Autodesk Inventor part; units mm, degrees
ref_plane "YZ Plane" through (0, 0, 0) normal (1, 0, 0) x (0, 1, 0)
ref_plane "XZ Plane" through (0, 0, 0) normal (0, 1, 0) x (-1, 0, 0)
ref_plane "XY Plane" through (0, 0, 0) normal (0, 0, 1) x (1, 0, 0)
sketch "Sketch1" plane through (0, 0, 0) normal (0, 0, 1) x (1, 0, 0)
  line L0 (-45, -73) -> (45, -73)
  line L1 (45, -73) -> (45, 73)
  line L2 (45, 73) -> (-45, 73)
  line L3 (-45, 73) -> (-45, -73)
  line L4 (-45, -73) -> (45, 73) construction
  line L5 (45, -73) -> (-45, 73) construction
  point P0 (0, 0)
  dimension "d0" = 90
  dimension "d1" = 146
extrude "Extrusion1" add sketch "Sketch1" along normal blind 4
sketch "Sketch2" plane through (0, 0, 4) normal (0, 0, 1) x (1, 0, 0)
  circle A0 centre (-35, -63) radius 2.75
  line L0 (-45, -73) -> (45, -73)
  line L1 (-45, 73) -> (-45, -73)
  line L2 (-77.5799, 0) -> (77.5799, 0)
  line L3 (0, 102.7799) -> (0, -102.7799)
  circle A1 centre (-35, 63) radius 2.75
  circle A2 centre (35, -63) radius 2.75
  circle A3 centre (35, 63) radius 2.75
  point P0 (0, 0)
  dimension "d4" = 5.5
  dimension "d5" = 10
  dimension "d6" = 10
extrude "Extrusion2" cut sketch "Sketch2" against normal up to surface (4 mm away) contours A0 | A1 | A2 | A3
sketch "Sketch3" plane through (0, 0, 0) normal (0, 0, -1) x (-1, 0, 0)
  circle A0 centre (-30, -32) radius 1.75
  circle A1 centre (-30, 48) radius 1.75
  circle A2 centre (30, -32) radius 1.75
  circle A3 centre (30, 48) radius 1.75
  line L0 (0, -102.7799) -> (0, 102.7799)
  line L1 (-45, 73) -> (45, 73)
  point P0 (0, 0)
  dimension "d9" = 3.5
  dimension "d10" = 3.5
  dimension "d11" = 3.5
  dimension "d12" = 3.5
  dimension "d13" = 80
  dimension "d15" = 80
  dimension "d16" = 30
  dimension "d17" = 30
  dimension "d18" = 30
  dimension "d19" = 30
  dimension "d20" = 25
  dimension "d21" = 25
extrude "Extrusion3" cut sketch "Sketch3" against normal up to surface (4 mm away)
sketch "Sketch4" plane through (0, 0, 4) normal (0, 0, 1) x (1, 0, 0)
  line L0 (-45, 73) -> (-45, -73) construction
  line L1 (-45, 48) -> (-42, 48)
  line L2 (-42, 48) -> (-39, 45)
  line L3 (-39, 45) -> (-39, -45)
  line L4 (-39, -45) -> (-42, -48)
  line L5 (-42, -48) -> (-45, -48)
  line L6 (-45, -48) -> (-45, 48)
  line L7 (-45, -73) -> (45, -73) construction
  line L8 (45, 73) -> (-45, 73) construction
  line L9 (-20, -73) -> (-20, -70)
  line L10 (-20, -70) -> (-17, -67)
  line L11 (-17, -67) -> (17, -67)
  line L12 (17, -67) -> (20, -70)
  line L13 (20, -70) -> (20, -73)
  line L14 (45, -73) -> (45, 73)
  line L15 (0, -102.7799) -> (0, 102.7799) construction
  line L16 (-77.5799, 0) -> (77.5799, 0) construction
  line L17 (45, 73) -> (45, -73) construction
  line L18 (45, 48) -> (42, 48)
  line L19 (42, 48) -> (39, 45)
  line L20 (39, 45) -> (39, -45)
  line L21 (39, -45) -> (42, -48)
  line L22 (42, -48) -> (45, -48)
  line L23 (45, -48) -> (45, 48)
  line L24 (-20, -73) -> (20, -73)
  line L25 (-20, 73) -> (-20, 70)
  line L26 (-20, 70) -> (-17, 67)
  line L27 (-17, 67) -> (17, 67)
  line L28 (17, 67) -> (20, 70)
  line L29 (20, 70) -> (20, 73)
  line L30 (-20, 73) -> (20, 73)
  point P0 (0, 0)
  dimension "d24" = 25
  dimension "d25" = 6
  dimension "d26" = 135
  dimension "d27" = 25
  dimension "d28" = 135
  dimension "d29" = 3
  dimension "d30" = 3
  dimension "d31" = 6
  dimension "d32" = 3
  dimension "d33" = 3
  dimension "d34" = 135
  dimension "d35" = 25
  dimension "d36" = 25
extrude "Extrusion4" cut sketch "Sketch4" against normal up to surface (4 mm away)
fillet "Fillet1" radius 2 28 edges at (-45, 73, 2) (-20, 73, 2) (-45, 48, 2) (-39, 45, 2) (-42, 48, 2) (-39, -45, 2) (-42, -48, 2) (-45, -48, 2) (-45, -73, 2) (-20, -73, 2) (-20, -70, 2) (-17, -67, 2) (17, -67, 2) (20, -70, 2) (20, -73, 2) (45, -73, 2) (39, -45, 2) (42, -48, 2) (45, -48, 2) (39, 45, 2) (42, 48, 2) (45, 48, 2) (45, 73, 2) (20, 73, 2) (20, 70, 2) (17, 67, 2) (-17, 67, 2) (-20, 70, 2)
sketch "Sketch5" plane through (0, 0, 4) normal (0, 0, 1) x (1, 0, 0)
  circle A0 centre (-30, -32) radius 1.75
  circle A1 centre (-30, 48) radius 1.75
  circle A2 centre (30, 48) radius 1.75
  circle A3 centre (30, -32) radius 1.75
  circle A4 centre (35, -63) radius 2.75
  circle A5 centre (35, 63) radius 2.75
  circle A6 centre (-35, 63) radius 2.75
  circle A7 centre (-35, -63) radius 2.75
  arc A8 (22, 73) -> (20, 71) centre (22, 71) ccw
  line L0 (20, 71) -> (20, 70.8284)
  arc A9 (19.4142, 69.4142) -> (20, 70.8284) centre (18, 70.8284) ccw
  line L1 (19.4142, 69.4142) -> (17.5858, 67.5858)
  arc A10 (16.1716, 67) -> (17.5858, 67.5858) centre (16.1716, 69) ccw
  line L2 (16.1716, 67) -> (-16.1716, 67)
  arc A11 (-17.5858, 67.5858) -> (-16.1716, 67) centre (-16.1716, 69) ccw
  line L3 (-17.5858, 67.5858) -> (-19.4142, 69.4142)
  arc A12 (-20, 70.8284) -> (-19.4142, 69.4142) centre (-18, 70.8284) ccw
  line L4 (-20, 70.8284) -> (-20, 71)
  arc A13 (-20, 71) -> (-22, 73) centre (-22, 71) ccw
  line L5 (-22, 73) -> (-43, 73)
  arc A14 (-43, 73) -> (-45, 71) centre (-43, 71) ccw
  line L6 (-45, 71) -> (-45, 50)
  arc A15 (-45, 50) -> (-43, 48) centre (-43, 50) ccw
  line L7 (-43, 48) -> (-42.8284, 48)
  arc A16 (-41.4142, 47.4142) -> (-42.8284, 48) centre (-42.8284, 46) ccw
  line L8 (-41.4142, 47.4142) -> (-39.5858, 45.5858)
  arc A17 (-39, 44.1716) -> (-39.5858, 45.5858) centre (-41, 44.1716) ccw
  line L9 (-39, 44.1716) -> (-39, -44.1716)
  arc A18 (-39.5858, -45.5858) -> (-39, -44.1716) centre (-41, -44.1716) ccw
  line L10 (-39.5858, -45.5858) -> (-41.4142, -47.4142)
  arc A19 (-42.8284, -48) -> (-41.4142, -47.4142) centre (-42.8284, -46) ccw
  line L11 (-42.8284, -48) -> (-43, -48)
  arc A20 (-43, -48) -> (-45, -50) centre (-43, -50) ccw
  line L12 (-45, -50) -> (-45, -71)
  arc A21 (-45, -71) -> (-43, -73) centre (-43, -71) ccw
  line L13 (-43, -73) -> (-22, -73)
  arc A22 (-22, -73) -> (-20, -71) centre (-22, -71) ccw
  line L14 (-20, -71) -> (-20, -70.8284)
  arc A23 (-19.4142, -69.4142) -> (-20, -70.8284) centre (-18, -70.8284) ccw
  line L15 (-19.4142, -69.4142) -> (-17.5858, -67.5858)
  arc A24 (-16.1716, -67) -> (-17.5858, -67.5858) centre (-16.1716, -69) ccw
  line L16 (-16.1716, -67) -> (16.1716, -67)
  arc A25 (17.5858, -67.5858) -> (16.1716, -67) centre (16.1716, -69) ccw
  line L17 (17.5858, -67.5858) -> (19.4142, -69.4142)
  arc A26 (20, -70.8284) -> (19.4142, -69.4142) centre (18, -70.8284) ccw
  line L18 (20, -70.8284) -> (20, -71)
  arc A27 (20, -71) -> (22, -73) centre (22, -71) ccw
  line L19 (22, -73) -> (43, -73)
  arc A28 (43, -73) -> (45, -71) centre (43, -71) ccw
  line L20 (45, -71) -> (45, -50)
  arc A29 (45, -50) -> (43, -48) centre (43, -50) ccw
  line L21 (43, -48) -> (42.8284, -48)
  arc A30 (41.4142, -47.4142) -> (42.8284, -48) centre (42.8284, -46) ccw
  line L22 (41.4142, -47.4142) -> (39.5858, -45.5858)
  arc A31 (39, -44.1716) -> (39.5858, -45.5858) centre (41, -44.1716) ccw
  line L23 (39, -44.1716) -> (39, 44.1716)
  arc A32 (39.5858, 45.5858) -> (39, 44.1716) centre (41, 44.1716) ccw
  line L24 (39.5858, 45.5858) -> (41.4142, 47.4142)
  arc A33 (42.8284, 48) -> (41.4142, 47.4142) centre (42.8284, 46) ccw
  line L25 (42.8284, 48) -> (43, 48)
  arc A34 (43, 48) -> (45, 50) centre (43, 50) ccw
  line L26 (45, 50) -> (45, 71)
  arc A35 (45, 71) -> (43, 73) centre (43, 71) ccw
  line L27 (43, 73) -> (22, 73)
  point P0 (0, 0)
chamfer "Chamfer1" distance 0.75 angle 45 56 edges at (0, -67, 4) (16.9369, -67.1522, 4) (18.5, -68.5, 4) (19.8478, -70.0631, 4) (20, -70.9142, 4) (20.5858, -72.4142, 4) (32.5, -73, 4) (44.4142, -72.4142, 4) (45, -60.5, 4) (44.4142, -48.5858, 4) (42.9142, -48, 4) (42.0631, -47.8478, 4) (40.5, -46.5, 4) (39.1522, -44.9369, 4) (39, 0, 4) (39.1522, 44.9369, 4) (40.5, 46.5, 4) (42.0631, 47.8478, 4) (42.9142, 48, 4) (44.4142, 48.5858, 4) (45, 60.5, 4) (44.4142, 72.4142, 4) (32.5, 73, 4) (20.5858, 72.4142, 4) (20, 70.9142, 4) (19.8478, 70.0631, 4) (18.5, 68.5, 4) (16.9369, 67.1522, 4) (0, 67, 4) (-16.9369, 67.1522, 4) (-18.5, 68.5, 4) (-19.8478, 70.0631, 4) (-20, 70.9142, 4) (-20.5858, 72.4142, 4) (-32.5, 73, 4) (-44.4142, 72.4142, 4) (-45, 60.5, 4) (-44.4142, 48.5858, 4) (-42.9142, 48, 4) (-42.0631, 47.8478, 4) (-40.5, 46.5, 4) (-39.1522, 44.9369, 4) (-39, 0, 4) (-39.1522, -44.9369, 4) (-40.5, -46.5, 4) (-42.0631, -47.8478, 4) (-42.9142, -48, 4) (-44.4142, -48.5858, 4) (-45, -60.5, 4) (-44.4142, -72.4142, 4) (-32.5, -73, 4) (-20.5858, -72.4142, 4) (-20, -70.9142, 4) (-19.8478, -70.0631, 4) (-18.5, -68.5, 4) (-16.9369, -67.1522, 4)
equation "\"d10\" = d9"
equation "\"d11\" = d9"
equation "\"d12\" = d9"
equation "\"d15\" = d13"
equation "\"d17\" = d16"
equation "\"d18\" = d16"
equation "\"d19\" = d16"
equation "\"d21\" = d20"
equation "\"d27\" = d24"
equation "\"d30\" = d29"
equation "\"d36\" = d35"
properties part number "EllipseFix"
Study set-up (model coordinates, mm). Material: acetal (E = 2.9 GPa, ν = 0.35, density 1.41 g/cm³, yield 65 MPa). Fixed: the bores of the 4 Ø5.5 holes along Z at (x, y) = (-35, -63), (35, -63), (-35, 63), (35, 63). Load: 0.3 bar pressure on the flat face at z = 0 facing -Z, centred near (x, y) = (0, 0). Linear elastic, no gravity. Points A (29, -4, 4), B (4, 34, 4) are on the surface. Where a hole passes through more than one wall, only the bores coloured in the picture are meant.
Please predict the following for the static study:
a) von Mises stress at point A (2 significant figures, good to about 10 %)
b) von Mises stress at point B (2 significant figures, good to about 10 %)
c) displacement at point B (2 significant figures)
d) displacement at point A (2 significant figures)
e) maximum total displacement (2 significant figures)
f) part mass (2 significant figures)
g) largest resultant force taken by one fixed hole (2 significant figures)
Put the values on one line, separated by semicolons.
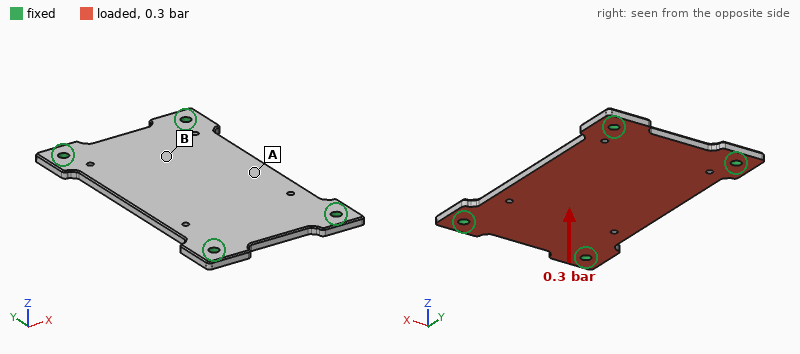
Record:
8.2 MPa; 3.3 MPa; 0.97 mm; 1.5 mm; 1.6 mm; 64 g; 86 N
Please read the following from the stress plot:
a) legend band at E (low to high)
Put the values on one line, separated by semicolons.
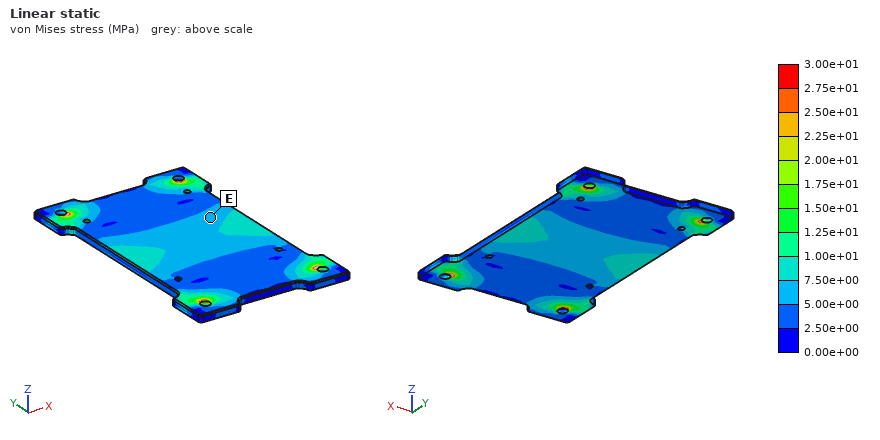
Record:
5.00e+00 to 7.50e+00 MPa
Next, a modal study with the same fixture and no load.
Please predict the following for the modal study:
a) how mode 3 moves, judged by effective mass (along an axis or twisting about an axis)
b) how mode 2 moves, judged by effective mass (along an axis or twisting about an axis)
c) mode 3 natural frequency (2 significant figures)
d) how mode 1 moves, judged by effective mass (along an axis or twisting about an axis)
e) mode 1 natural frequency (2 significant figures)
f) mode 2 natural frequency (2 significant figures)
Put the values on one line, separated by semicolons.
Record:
twisting about X; twisting about Y; 870 Hz; along Z; 330 Hz; 570 Hz
